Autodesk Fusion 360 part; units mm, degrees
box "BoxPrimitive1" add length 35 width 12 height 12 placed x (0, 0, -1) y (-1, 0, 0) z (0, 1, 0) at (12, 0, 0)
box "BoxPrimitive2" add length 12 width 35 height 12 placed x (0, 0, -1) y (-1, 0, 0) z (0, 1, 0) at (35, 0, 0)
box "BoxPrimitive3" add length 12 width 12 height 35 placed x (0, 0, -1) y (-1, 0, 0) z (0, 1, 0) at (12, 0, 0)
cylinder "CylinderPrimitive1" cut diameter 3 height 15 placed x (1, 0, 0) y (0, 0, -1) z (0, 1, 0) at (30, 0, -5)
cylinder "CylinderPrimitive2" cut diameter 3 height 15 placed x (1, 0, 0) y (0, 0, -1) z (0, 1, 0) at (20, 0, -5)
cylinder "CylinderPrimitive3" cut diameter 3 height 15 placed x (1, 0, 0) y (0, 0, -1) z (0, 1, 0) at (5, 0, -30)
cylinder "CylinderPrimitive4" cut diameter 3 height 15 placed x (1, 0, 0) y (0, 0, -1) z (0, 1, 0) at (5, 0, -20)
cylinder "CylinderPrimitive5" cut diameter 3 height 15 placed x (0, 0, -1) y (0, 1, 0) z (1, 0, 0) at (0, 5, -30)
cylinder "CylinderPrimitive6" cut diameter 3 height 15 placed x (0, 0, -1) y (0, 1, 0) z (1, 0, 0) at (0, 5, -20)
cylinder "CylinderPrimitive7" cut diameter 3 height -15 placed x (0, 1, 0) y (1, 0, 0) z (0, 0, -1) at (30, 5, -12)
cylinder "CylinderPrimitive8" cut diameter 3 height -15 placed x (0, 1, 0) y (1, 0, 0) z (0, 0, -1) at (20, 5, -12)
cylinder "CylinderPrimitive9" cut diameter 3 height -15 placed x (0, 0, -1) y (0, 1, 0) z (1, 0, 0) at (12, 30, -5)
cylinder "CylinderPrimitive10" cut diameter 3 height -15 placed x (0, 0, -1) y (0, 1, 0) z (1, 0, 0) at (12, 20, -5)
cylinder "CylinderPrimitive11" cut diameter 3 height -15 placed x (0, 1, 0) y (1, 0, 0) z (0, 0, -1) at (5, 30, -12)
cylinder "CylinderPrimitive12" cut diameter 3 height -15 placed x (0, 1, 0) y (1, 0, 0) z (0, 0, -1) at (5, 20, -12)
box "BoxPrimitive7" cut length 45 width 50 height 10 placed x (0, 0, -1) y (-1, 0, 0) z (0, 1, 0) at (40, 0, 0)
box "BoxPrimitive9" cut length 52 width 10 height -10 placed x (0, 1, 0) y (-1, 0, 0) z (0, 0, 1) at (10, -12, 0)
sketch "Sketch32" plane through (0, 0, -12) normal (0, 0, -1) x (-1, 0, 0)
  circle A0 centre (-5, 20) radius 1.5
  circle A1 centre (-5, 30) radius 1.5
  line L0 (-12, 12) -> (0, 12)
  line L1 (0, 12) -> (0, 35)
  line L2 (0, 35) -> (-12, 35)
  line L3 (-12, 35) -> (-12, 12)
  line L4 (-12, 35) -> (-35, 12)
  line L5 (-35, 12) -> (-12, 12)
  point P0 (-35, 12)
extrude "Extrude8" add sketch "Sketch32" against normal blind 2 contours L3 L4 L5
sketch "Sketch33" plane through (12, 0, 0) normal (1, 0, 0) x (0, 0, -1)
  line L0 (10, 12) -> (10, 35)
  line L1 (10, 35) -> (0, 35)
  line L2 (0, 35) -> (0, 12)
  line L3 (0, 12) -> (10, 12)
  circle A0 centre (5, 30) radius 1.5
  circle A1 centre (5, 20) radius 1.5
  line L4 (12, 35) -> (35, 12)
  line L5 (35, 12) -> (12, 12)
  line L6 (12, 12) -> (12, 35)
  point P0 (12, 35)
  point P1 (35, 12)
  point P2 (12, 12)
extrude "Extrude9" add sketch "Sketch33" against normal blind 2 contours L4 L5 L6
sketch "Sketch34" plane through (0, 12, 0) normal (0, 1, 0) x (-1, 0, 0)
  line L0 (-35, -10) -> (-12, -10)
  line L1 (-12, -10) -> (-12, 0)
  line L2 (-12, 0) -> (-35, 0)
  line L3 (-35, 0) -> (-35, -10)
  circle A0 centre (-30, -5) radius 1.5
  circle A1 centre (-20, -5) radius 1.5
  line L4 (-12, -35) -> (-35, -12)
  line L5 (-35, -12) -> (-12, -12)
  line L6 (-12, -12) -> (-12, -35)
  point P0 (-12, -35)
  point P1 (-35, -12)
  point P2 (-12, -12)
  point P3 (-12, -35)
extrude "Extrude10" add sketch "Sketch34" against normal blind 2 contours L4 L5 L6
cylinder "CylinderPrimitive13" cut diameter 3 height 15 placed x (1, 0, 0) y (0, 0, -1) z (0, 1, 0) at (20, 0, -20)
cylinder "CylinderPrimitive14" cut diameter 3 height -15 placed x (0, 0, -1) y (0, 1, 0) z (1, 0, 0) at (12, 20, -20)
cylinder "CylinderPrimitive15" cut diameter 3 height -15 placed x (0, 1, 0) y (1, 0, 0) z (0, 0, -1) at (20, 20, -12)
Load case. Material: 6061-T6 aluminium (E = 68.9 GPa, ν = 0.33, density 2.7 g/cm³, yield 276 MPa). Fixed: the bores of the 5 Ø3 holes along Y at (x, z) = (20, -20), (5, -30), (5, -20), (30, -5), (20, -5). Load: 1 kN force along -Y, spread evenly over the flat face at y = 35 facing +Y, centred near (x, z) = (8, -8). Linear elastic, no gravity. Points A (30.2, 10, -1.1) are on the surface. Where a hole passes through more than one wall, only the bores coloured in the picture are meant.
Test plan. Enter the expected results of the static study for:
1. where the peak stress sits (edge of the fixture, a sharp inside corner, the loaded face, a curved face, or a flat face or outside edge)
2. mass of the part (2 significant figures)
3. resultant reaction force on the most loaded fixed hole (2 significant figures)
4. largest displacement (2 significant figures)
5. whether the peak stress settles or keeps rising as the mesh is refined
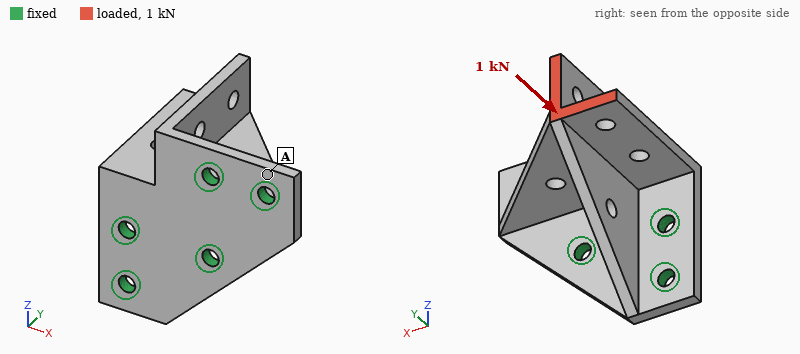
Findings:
edge of the fixture
9.8 g
690 N
0.14 mm
keeps rising
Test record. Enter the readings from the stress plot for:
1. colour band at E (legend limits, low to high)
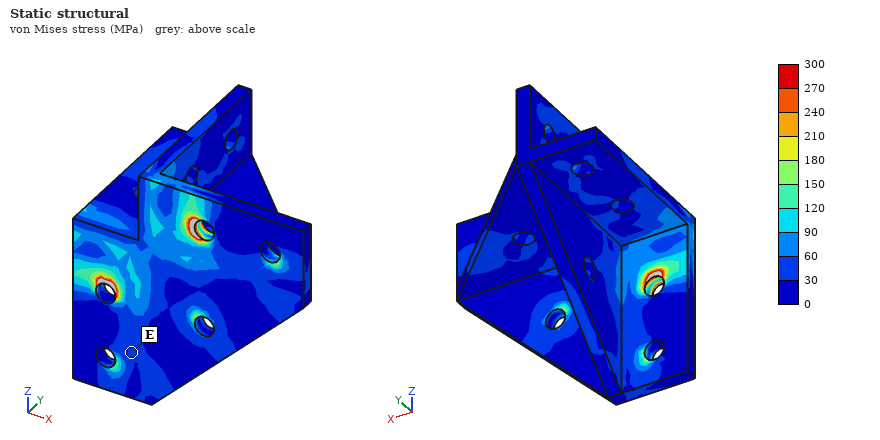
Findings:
30 to 60 MPa
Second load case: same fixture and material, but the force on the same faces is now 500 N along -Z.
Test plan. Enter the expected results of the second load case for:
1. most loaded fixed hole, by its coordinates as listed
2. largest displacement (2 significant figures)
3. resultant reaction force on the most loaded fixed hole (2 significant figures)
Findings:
(20, -5)
0.28 mm
530 N
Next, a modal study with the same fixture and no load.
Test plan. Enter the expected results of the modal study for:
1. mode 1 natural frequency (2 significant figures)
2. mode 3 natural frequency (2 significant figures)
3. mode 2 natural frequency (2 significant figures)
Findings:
6700 Hz
14 kHz
8500 Hz
